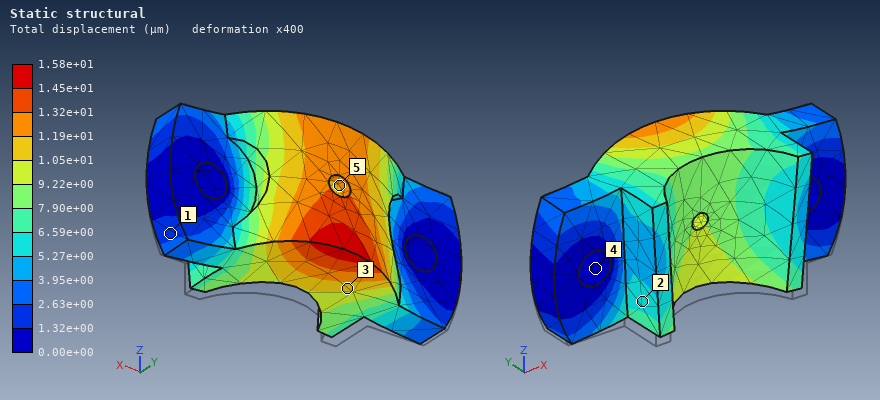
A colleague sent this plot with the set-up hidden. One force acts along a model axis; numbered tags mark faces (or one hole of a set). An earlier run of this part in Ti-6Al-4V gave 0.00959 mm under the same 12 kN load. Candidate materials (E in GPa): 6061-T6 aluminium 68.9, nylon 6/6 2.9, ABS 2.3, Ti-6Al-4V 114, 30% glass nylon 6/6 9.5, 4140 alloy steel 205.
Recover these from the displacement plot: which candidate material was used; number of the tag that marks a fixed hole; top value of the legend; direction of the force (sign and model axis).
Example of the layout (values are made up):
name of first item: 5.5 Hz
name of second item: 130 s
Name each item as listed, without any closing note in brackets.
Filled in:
which candidate material was used: 6061-T6 aluminium
number of the tag that marks a fixed hole: 4
top value of the legend: 1.58e+01 µm
direction of the force: +Z
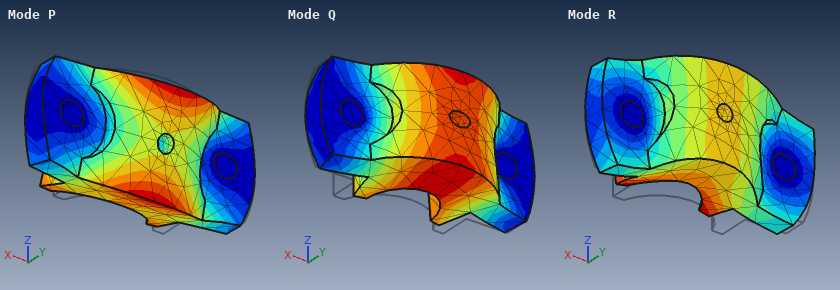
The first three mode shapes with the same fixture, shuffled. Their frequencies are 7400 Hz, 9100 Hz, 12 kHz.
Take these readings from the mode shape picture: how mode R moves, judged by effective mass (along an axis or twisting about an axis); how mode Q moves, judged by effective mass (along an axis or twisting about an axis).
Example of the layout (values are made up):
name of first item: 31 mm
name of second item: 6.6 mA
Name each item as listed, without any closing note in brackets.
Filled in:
how mode R moves, judged by effective mass: along Z
how mode Q moves, judged by effective mass: along Y
